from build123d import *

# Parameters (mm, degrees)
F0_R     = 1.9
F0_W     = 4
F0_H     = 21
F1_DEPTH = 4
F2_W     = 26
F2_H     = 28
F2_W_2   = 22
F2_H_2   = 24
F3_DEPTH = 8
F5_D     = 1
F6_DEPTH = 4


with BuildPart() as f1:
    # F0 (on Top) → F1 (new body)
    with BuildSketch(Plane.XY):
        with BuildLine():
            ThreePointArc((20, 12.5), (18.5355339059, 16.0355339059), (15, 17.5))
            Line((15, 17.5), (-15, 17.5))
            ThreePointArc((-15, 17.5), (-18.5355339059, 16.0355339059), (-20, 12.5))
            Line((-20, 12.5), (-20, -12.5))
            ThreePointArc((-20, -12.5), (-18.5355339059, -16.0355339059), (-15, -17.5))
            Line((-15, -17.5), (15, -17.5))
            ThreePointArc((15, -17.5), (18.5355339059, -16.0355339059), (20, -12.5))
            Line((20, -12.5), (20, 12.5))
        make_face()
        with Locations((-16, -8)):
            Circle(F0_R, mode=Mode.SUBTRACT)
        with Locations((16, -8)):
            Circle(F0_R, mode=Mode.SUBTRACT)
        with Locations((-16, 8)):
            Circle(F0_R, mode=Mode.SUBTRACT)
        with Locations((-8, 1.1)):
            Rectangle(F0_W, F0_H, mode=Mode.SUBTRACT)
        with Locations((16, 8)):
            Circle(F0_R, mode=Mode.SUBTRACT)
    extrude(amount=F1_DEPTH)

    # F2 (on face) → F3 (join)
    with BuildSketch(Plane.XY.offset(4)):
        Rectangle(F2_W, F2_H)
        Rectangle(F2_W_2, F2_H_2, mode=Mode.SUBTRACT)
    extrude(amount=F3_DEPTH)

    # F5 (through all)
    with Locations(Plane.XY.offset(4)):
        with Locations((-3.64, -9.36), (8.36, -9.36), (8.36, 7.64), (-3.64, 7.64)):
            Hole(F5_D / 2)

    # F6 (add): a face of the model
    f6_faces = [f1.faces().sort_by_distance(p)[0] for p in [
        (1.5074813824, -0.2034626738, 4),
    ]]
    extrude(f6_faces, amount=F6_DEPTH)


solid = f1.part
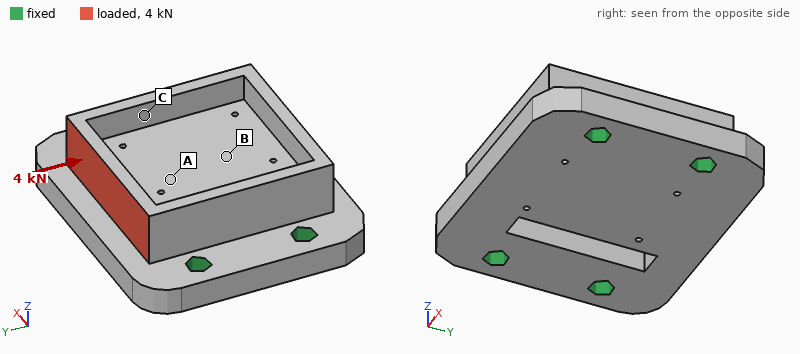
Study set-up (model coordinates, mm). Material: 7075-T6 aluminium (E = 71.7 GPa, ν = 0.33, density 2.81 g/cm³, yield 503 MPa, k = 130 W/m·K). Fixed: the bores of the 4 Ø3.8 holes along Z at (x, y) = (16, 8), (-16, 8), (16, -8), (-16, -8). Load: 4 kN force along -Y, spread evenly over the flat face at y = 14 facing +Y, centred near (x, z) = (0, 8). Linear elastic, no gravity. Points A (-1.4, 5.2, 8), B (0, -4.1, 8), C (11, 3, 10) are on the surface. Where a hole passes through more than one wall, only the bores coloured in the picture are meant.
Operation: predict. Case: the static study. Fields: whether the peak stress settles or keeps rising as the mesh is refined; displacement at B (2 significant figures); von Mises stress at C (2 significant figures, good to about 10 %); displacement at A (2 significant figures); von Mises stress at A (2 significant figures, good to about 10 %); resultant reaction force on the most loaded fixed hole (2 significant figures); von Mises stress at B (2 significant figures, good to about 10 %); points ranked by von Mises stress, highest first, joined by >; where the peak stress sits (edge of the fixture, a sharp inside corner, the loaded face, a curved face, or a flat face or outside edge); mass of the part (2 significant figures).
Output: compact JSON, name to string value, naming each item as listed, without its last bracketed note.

{"whether the peak stress settles or keeps rising as the mesh is refined": "keeps rising", "displacement at B": "11 µm", "von Mises stress at C": "33 MPa", "displacement at A": "15 µm", "von Mises stress at A": "55 MPa", "resultant reaction force on the most loaded fixed hole": "1.7 kN", "von Mises stress at B": "16 MPa", "points ranked by von Mises stress, highest first, joined by >": "A > C > B", "where the peak stress sits": "edge of the fixture", "mass of the part": "23 g"}
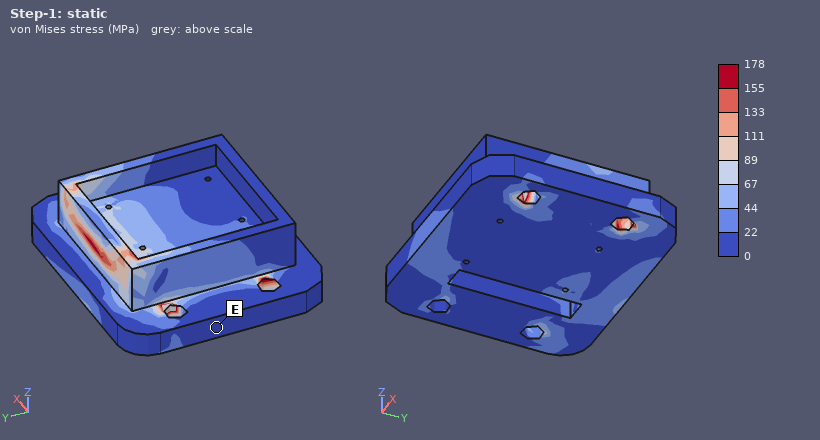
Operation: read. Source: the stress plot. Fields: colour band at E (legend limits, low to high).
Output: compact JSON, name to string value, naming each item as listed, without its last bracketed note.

{"colour band at E": "0 to 22 MPa"}
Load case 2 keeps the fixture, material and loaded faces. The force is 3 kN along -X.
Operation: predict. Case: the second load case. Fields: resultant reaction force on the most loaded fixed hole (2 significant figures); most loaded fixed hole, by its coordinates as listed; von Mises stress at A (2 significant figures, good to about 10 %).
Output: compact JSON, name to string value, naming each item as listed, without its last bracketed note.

{"resultant reaction force on the most loaded fixed hole": "1.9 kN", "most loaded fixed hole, by its coordinates as listed": "(16, 8)", "von Mises stress at A": "14 MPa"}
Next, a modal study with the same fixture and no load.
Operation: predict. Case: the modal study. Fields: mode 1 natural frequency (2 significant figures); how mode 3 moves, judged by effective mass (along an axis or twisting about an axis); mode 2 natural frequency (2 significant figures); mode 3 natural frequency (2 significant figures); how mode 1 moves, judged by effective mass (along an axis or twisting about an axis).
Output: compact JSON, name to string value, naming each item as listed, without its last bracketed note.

{"mode 1 natural frequency": "19 kHz", "how mode 3 moves, judged by effective mass": "along Y", "mode 2 natural frequency": "20 kHz", "mode 3 natural frequency": "28 kHz", "how mode 1 moves, judged by effective mass": "along Z"}
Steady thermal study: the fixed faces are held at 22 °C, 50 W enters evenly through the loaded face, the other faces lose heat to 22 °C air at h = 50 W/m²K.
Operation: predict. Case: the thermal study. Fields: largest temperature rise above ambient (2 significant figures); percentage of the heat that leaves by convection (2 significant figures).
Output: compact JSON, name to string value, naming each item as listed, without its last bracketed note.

{"largest temperature rise above ambient": "41 K", "percentage of the heat that leaves by convection": "4.2 %"}
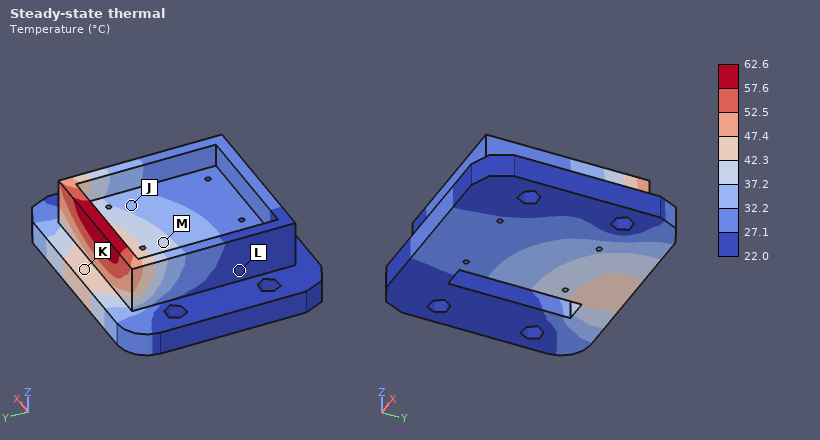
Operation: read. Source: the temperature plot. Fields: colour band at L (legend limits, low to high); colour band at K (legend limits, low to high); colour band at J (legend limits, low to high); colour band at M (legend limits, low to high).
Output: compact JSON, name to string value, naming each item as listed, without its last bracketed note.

{"colour band at L": "22.0 to 27.1 °C", "colour band at K": "42.3 to 47.4 °C", "colour band at J": "32.2 to 37.2 °C", "colour band at M": "37.2 to 42.3 °C"}
